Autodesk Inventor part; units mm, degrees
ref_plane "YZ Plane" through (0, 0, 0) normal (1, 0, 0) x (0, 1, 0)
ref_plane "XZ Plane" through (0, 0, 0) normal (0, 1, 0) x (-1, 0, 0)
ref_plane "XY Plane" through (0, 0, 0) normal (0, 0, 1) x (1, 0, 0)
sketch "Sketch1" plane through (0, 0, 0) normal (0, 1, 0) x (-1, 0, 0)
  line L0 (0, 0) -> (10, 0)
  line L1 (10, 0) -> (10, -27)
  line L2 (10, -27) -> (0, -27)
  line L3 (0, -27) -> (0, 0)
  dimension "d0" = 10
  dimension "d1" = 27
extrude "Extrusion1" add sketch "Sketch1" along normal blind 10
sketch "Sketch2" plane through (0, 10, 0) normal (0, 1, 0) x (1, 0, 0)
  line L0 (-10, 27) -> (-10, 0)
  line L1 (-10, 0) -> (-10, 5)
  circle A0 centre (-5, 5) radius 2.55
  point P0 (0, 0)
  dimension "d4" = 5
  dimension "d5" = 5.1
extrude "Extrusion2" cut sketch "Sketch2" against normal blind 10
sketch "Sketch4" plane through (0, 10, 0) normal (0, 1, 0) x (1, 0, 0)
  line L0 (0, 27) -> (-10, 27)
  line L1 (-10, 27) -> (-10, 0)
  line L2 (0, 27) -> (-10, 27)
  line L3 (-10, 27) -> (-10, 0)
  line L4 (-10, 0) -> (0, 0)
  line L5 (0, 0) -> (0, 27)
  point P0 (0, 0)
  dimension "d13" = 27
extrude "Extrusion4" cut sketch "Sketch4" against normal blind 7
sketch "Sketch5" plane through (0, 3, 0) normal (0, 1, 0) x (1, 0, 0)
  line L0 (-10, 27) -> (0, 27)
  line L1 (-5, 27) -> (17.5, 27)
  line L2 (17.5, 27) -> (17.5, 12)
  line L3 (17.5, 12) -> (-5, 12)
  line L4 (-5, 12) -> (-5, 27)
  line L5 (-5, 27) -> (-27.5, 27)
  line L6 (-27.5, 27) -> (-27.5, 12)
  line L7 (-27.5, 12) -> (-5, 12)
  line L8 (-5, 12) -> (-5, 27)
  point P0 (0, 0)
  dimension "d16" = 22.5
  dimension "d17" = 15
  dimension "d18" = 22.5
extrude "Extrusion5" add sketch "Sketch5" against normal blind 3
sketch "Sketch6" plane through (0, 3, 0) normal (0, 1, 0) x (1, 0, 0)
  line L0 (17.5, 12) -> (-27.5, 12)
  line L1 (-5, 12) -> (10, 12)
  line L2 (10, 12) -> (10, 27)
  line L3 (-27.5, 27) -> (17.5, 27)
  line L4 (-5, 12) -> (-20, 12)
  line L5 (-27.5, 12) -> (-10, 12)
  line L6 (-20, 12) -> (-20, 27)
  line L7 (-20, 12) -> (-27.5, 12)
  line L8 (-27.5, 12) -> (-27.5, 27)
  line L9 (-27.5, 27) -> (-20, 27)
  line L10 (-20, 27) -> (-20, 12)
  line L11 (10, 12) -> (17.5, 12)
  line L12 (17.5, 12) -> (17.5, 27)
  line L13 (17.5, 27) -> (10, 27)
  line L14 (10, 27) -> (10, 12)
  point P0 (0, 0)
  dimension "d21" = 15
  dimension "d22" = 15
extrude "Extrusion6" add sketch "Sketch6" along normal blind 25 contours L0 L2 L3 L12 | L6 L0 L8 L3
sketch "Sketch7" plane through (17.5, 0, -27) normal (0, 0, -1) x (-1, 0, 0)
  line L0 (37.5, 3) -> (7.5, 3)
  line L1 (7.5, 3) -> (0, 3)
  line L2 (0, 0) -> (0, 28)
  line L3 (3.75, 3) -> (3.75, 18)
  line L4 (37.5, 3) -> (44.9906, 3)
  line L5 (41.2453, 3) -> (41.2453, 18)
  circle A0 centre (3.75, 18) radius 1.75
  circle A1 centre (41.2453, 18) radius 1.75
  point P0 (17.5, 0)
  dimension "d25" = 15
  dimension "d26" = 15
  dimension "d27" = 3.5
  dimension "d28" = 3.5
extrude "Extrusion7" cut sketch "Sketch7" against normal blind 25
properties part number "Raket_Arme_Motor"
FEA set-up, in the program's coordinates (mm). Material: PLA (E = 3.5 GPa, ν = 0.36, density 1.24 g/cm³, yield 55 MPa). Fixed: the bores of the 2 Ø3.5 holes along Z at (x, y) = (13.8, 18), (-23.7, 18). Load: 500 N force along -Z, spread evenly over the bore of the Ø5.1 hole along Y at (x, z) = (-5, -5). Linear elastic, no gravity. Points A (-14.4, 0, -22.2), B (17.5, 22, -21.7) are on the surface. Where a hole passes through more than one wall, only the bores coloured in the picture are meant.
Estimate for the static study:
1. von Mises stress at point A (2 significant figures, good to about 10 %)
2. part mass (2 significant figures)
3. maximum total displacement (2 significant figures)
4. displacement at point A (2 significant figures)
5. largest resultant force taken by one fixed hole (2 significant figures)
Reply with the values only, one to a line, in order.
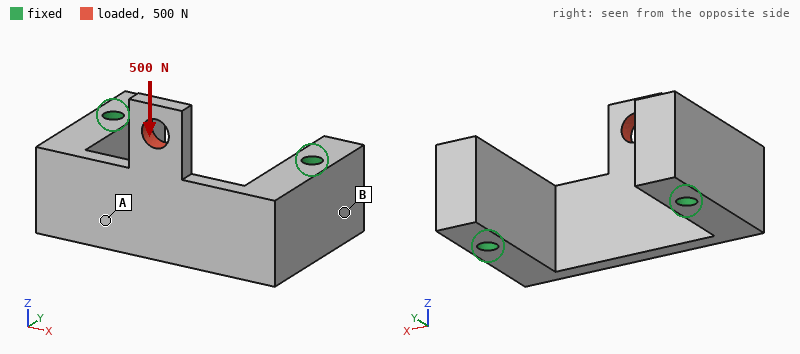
12 MPa
9.5 g
0.33 mm
0.18 mm
250 N
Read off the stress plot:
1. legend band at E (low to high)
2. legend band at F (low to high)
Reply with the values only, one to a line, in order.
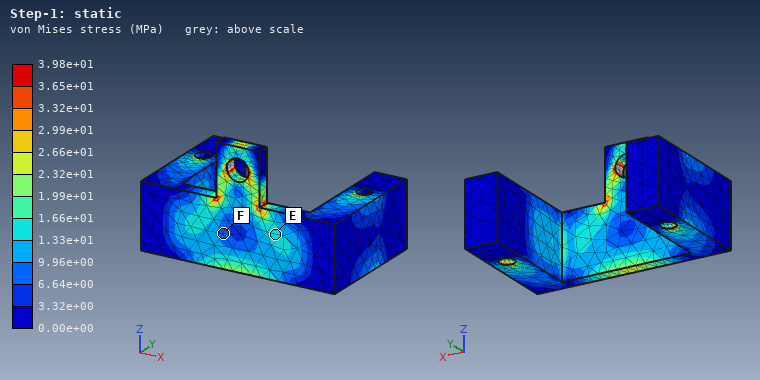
1.33e+01 to 1.66e+01 MPa
6.64e+00 to 9.96e+00 MPa
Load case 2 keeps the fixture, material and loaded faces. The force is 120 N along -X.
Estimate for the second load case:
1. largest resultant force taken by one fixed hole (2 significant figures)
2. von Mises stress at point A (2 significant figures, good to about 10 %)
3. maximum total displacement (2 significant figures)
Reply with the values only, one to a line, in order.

76 N
2.9 MPa
0.25 mm
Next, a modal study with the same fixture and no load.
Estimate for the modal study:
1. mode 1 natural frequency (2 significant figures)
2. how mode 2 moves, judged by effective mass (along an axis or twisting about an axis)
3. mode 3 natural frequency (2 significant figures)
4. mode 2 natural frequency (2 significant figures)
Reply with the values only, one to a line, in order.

2200 Hz
along X
4700 Hz
3800 Hz
